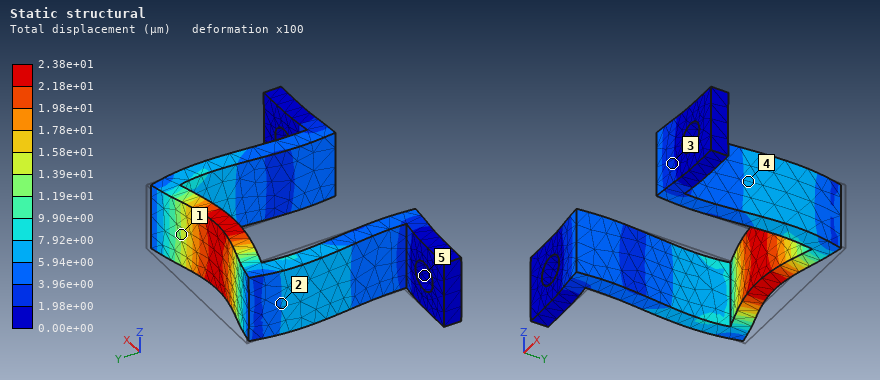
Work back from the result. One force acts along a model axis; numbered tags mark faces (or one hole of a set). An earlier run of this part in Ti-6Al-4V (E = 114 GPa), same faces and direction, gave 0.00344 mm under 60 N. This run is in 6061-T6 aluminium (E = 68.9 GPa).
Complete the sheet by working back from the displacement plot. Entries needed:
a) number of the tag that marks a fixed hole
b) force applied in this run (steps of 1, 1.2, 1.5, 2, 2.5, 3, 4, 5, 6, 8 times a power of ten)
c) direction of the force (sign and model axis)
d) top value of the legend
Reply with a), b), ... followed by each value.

a) 5
b) 250 N
c) -Y
d) 2.38e+01 µm
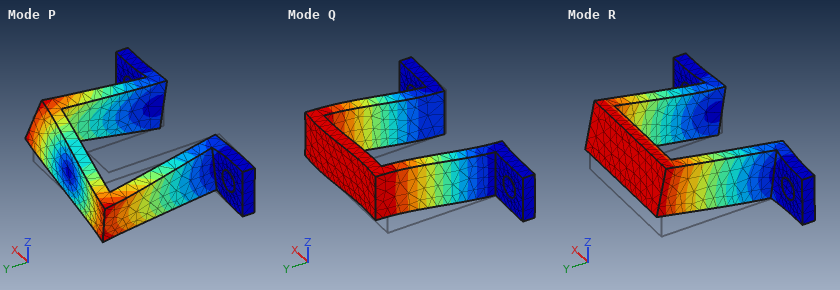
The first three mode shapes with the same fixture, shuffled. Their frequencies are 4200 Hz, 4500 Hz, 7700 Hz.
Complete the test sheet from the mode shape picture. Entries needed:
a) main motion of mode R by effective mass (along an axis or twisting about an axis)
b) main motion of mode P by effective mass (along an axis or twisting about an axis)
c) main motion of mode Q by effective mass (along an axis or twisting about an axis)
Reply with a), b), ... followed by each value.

a) along Z
b) twisting about Y
c) along X
